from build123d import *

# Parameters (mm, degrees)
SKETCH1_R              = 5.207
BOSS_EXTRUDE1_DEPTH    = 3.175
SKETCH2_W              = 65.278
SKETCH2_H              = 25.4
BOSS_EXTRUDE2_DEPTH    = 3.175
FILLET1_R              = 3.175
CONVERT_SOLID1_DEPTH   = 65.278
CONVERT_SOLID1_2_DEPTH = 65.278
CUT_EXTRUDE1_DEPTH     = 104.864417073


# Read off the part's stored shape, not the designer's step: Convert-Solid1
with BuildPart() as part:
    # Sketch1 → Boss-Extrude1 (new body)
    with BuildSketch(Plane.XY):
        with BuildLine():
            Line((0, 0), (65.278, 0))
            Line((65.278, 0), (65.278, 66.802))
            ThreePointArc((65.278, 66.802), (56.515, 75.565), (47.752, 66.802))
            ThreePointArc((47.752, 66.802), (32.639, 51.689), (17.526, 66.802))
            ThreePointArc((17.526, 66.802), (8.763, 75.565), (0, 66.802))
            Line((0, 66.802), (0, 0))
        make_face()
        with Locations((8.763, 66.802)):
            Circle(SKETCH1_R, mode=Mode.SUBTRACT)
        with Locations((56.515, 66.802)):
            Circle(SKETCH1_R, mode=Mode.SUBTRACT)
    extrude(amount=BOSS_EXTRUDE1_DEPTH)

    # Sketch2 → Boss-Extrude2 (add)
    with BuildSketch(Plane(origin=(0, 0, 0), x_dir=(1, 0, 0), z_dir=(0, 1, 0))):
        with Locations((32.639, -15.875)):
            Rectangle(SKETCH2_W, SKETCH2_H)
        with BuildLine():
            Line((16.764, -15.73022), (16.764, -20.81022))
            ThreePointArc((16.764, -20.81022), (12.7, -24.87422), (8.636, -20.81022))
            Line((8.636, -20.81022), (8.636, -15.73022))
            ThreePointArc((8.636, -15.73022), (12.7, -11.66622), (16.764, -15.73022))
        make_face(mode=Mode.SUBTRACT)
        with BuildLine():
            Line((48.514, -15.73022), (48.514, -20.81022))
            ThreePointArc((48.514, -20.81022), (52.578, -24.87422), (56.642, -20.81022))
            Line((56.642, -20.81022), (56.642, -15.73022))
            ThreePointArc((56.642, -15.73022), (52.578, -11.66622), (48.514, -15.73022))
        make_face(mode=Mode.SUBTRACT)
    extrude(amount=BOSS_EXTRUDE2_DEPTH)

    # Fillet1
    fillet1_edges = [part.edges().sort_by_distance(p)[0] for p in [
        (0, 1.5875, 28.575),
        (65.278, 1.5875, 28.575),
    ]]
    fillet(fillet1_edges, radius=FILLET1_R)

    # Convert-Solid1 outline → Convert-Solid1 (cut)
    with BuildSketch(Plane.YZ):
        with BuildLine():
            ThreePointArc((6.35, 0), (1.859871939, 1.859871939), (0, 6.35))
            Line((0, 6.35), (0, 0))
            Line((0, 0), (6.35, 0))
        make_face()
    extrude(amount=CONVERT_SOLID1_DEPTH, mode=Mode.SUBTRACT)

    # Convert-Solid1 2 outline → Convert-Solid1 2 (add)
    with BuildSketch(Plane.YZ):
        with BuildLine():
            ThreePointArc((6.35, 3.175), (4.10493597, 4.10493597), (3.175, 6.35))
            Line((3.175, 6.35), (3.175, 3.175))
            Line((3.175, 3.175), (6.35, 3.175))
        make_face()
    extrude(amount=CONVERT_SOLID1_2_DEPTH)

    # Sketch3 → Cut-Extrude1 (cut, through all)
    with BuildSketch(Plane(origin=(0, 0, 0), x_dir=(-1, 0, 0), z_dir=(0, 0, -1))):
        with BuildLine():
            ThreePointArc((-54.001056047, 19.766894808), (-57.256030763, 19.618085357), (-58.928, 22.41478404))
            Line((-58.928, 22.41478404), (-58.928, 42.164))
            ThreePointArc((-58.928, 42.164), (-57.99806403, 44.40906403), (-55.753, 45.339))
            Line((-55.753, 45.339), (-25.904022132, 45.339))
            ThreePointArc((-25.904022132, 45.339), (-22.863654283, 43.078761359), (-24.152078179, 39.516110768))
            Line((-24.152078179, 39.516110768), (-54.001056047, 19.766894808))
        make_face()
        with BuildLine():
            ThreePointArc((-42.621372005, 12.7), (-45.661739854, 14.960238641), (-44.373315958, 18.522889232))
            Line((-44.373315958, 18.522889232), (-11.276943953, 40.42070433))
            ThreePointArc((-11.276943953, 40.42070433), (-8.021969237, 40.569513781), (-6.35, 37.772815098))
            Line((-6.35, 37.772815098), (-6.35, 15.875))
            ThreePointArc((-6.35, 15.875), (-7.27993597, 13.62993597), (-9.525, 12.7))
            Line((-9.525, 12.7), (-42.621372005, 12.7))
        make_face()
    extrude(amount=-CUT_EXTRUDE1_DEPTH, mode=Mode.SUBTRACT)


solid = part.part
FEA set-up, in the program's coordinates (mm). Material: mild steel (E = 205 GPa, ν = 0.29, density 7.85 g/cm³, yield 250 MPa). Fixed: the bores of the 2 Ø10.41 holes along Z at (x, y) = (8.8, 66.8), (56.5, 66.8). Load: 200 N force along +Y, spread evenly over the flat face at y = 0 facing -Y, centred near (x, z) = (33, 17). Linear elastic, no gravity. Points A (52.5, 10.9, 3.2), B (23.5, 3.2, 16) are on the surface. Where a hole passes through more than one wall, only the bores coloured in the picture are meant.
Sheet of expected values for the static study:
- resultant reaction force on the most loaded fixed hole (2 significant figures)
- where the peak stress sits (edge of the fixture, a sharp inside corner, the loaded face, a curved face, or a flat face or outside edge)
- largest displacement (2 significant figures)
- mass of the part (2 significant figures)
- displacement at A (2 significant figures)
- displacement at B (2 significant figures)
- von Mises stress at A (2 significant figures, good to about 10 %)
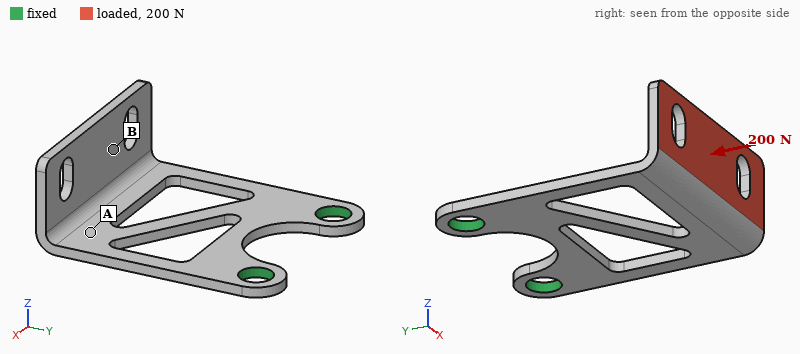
110 N
a curved face
0.61 mm
100 g
0.30 mm
0.46 mm
53 MPa
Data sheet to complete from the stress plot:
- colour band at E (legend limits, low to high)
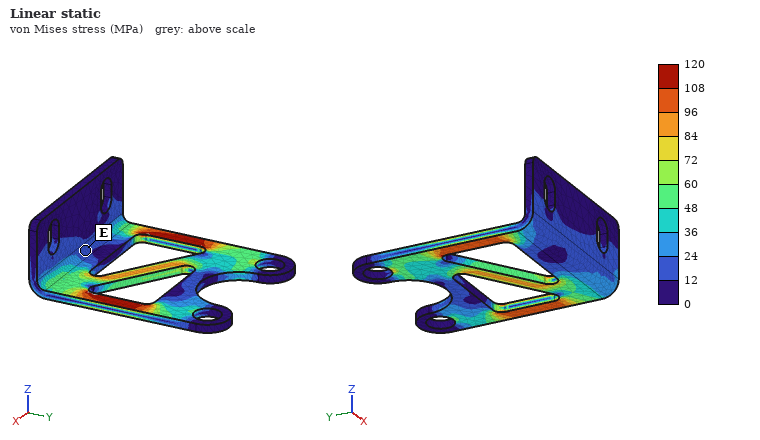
12 to 24 MPa
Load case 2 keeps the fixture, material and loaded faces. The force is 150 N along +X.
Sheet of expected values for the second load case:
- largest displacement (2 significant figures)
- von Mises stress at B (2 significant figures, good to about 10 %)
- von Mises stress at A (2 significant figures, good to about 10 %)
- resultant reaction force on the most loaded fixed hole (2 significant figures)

0.14 mm
8.2 MPa
27 MPa
180 N
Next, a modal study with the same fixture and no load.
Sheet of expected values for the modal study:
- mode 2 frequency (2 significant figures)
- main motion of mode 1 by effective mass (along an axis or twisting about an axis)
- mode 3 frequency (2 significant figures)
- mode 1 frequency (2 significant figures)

770 Hz
along Z
1400 Hz
290 Hz
